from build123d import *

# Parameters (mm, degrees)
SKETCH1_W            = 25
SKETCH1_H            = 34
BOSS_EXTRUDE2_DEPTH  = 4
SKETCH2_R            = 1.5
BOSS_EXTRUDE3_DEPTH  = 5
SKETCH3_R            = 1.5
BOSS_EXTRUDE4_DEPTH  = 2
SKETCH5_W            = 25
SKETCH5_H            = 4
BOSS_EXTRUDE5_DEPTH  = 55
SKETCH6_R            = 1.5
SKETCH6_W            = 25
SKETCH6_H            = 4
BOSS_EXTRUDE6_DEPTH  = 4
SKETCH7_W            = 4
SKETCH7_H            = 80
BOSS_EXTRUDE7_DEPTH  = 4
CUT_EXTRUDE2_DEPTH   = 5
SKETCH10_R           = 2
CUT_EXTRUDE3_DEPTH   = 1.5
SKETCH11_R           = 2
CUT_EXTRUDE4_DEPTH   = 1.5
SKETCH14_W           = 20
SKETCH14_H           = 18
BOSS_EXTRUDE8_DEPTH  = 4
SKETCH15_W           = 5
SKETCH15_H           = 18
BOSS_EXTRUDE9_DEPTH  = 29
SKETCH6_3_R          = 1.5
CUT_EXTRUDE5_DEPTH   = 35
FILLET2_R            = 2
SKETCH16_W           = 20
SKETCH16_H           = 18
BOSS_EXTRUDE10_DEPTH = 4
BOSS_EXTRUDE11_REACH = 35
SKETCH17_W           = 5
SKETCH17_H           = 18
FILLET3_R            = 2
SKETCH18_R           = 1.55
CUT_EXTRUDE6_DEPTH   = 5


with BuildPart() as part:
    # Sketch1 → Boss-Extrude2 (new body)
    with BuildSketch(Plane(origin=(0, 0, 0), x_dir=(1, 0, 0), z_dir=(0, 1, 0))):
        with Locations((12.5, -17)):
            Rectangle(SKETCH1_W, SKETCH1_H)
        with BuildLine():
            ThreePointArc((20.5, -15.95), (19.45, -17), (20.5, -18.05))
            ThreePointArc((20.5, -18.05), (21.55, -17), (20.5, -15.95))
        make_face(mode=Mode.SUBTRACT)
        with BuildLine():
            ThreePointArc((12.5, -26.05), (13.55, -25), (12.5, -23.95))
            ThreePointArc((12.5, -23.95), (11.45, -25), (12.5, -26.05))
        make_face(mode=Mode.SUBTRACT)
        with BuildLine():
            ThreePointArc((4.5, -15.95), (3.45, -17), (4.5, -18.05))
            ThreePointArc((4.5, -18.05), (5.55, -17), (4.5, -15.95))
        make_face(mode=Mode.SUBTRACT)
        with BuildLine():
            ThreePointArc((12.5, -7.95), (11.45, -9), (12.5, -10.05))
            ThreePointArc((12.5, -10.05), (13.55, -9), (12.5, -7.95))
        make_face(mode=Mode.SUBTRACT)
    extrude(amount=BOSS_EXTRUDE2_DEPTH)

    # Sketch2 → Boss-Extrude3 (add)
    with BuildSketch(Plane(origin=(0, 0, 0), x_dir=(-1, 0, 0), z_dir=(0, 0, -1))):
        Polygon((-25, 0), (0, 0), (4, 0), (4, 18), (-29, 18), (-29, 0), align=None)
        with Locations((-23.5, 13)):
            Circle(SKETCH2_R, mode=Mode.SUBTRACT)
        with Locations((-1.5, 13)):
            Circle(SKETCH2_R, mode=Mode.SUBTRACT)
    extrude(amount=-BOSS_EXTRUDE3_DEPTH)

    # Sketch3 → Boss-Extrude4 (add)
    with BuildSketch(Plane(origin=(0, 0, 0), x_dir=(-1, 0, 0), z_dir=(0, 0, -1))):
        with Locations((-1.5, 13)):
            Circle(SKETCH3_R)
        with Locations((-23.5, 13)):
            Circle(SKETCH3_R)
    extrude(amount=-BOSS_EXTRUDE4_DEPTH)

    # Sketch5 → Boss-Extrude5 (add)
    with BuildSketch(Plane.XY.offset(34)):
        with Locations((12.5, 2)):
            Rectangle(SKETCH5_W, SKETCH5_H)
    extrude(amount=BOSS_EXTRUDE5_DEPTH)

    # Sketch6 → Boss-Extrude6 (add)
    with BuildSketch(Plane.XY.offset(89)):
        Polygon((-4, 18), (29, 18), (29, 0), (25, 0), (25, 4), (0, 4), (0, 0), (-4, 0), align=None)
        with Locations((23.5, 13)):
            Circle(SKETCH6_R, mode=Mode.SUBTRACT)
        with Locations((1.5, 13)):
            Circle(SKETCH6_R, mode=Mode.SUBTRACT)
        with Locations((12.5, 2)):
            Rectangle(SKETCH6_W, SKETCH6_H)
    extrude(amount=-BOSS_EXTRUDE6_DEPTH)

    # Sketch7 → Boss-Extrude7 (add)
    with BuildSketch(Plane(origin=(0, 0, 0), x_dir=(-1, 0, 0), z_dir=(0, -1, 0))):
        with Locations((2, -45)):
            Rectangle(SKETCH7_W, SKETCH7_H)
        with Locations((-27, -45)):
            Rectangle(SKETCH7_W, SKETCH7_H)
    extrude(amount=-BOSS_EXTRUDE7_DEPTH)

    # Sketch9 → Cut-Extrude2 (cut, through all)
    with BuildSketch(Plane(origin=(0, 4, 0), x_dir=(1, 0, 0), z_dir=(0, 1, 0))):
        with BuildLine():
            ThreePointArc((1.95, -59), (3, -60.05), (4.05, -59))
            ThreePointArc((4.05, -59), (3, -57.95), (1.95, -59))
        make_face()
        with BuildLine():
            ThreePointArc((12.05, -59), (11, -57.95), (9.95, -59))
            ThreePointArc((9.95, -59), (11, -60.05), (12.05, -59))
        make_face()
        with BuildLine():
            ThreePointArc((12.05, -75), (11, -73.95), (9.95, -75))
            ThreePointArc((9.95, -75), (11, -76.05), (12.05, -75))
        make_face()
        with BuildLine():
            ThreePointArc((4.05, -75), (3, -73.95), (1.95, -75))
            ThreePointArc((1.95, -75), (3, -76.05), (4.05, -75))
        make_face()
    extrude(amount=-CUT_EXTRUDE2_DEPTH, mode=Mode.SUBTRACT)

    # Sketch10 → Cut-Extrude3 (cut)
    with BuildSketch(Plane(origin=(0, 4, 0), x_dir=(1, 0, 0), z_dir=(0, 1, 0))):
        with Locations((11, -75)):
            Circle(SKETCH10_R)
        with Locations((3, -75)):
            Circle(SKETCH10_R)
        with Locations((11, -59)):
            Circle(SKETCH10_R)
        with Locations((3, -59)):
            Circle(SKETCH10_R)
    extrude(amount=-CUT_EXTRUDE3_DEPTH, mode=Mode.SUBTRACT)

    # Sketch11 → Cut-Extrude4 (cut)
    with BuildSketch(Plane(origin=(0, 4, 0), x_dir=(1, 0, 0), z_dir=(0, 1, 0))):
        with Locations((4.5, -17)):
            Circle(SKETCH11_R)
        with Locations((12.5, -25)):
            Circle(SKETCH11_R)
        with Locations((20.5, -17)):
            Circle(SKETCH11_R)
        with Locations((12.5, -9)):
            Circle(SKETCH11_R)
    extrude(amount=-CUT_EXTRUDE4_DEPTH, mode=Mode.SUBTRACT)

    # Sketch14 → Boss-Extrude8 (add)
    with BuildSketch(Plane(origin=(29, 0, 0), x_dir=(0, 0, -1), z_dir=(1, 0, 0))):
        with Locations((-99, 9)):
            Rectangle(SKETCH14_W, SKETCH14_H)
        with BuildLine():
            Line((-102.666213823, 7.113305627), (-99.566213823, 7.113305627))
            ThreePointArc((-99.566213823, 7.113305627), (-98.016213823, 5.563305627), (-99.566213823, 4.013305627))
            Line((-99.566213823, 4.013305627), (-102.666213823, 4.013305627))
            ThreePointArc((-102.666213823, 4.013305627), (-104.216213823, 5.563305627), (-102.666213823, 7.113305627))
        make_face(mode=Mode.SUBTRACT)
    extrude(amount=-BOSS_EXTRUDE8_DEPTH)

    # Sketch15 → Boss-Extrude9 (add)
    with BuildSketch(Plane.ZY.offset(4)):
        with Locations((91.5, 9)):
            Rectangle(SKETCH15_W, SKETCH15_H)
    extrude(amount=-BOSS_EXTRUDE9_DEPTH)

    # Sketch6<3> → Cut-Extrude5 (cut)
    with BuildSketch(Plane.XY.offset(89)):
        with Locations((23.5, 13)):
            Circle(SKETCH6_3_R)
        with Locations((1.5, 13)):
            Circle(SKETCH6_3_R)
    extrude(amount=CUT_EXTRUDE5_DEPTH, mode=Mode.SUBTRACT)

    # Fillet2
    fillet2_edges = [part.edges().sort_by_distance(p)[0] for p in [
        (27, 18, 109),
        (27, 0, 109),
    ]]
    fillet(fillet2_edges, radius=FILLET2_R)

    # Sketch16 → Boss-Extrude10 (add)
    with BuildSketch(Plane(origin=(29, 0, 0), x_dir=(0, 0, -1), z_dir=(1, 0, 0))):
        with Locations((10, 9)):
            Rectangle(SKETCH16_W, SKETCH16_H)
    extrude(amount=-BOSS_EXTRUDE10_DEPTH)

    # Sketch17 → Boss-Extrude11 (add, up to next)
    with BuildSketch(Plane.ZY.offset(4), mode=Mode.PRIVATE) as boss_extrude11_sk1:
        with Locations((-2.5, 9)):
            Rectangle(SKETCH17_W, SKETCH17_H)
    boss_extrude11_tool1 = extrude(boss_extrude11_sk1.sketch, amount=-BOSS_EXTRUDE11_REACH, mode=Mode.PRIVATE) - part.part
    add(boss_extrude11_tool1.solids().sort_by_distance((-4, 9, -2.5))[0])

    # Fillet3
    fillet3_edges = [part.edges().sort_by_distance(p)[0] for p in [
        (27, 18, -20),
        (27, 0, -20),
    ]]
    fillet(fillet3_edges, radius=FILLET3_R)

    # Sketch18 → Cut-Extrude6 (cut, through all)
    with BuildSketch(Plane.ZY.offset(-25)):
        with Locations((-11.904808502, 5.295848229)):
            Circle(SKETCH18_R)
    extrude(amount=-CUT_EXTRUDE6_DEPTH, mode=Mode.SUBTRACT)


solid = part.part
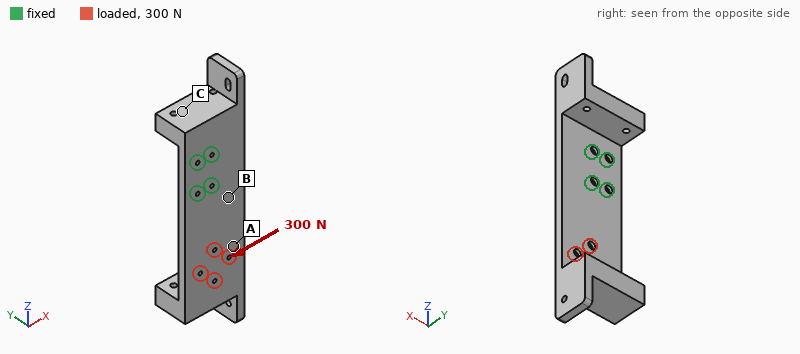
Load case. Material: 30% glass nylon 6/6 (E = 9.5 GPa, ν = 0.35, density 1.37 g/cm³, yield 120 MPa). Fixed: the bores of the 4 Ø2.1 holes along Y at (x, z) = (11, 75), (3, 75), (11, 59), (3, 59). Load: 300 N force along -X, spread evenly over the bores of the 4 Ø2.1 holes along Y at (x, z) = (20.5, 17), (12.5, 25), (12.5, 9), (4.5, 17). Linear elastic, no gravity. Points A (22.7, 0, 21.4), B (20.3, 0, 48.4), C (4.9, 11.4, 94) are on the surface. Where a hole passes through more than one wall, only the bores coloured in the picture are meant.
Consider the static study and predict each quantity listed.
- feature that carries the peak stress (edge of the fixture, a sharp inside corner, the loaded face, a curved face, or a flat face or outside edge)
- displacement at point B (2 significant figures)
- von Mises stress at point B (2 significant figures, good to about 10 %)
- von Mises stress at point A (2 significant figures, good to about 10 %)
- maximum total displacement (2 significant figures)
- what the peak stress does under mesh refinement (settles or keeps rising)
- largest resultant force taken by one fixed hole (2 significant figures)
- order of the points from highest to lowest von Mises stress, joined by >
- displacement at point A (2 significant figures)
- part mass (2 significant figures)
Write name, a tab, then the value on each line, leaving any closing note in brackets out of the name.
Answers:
feature that carries the peak stress	edge of the fixture
displacement at point B	0.055 mm
von Mises stress at point B	8.0 MPa
von Mises stress at point A	5.1 MPa
maximum total displacement	0.36 mm
what the peak stress does under mesh refinement	keeps rising
largest resultant force taken by one fixed hole	560 N
order of the points from highest to lowest von Mises stress, joined by >	B > A > C
displacement at point A	0.18 mm
part mass	32 g
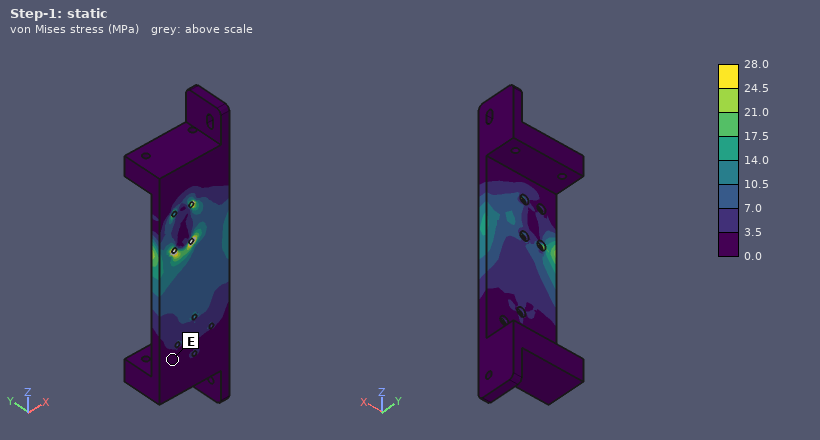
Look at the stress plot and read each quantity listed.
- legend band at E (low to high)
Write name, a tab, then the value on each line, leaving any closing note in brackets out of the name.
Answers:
legend band at E	0.0 to 3.5 MPa
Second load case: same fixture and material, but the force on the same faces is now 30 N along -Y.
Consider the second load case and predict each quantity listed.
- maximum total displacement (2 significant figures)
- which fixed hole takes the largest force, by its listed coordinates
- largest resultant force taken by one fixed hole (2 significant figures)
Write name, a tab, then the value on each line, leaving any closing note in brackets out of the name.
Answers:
maximum total displacement	1.3 mm
which fixed hole takes the largest force, by its listed coordinates	(11, 59)
largest resultant force taken by one fixed hole	85 N
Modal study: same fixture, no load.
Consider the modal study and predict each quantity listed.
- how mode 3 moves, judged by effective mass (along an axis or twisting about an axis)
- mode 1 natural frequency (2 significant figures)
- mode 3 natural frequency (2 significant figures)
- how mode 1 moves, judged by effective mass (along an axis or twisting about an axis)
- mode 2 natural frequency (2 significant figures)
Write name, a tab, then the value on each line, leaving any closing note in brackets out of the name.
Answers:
how mode 3 moves, judged by effective mass	along Y
mode 1 natural frequency	200 Hz
mode 3 natural frequency	1000 Hz
how mode 1 moves, judged by effective mass	along Y
mode 2 natural frequency	720 Hz
